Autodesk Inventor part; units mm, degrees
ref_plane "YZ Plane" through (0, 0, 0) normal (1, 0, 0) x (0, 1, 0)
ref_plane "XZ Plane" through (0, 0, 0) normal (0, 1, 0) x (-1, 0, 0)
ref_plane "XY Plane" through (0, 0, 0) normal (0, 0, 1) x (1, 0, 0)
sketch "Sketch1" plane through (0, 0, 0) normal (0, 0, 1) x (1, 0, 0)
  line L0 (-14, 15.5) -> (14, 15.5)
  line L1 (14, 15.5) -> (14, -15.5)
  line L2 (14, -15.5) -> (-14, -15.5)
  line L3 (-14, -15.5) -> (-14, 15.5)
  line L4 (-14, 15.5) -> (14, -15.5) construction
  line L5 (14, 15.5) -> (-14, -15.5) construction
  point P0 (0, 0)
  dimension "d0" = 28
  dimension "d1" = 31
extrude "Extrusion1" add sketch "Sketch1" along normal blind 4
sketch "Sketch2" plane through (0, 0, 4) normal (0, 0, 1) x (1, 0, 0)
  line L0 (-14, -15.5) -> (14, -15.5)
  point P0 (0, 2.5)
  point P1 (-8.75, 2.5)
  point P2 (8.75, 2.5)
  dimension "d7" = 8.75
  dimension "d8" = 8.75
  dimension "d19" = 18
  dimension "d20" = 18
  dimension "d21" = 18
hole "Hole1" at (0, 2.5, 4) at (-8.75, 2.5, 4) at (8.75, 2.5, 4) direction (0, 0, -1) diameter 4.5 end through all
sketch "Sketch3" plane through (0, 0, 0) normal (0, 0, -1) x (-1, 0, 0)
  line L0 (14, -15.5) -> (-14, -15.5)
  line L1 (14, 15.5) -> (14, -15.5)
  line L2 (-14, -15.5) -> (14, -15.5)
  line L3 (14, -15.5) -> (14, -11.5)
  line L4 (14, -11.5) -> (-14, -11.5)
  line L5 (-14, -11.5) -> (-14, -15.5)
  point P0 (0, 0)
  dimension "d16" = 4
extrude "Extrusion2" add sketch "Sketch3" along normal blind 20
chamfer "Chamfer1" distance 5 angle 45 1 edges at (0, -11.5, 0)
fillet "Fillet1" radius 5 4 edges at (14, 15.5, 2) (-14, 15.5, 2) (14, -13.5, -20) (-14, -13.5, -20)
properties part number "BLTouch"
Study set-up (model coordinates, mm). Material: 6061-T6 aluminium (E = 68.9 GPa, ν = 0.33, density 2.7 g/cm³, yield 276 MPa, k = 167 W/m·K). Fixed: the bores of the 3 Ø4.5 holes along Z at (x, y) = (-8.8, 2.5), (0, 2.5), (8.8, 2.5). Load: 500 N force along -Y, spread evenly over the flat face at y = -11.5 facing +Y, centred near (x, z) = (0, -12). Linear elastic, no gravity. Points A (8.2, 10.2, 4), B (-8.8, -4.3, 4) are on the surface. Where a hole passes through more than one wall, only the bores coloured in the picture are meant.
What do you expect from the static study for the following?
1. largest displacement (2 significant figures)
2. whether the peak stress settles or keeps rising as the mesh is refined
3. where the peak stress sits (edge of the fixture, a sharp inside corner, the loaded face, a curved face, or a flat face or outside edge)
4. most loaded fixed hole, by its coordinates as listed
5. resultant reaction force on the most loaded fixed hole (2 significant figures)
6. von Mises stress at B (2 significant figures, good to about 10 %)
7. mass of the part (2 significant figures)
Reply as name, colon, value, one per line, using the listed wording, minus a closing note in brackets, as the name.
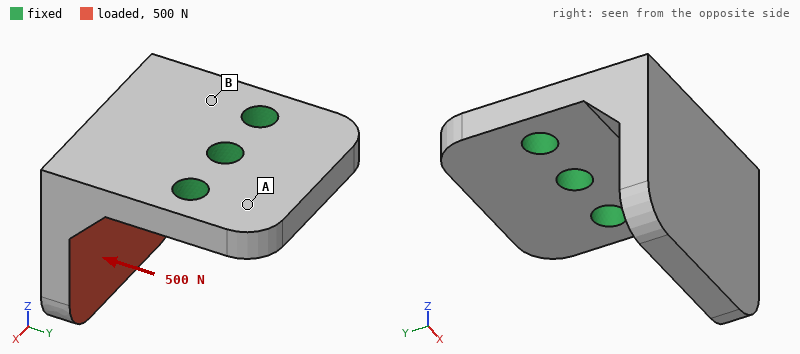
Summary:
largest displacement: 0.20 mm
whether the peak stress settles or keeps rising as the mesh is refined: keeps rising
where the peak stress sits: edge of the fixture
most loaded fixed hole, by its coordinates as listed: (0, 2.5)
resultant reaction force on the most loaded fixed hole: 200 N
von Mises stress at B: 81 MPa
mass of the part: 16 g
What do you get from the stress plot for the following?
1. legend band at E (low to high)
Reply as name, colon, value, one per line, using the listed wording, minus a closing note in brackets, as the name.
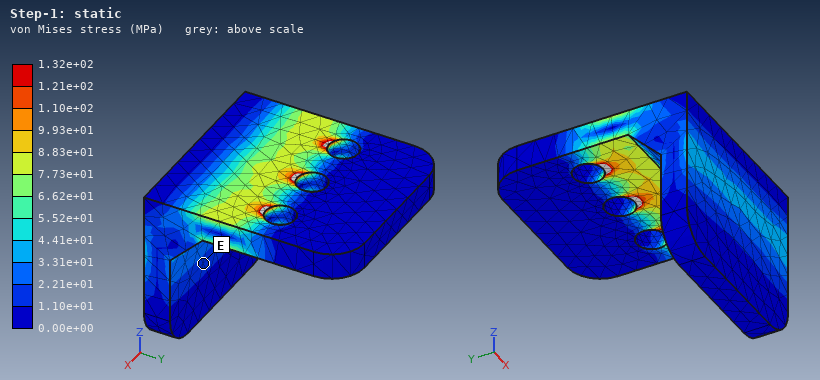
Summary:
legend band at E: 1.10e+01 to 2.21e+01 MPa
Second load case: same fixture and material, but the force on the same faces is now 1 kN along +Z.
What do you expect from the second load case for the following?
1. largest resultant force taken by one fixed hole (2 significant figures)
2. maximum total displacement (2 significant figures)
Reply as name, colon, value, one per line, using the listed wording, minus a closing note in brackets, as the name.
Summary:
largest resultant force taken by one fixed hole: 350 N
maximum total displacement: 0.16 mm
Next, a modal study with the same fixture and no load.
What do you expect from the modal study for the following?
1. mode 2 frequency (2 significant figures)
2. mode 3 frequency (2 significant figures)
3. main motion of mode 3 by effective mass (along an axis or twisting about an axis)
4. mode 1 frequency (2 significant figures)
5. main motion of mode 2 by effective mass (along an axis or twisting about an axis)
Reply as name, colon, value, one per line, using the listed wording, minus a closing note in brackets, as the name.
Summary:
mode 2 frequency: 7500 Hz
mode 3 frequency: 13 kHz
main motion of mode 3 by effective mass: along Z
mode 1 frequency: 3800 Hz
main motion of mode 2 by effective mass: along X
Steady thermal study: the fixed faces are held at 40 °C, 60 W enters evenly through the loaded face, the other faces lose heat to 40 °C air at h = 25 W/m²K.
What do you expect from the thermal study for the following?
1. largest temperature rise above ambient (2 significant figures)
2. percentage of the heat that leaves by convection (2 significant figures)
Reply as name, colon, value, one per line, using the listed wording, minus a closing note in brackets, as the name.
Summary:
largest temperature rise above ambient: 72 K
percentage of the heat that leaves by convection: 3.2 %
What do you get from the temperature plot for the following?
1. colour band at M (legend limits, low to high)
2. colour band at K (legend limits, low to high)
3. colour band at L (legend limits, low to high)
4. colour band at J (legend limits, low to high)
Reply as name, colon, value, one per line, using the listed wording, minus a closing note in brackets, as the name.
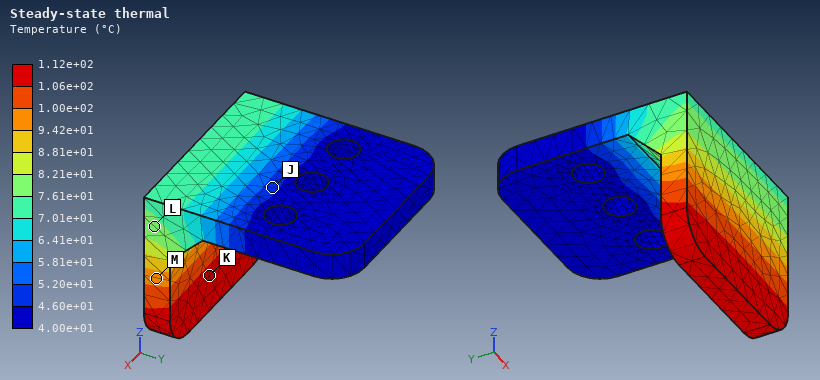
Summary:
colour band at M: 9.42e+01 to 1.00e+02 °C
colour band at K: 1.06e+02 to 1.12e+02 °C
colour band at L: 7.61e+01 to 8.21e+01 °C
colour band at J: 4.60e+01 to 5.20e+01 °C
